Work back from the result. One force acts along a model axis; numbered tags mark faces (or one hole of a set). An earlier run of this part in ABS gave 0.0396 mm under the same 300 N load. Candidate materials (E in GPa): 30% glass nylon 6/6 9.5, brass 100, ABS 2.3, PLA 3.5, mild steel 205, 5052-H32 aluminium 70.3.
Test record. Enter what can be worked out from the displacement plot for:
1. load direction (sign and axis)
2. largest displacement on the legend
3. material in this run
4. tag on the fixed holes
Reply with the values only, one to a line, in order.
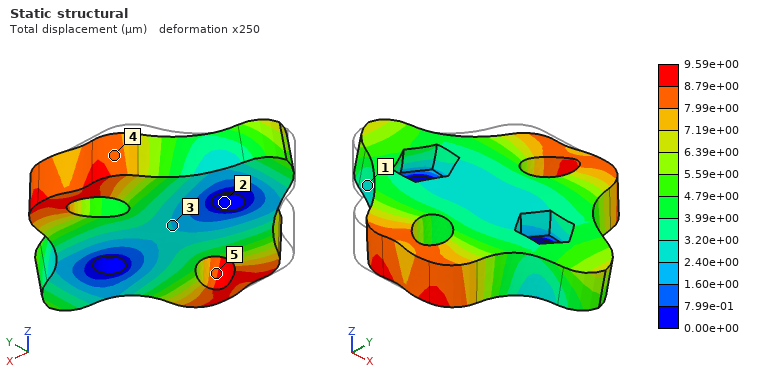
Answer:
+X
9.59e+00 µm
30% glass nylon 6/6
2
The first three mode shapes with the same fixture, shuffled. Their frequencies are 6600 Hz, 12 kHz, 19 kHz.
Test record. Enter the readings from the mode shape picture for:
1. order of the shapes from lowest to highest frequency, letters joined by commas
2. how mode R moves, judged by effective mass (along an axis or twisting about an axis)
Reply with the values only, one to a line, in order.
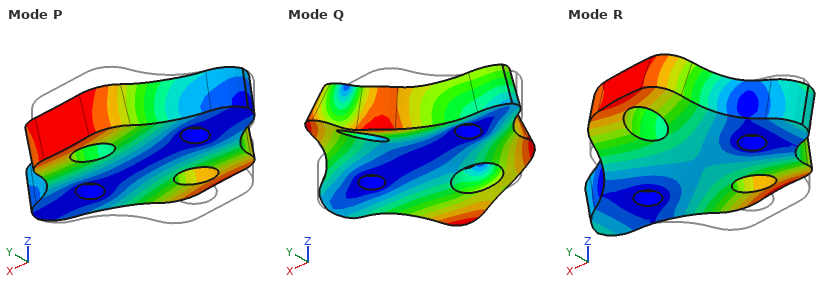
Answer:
P, R, Q
along Z
